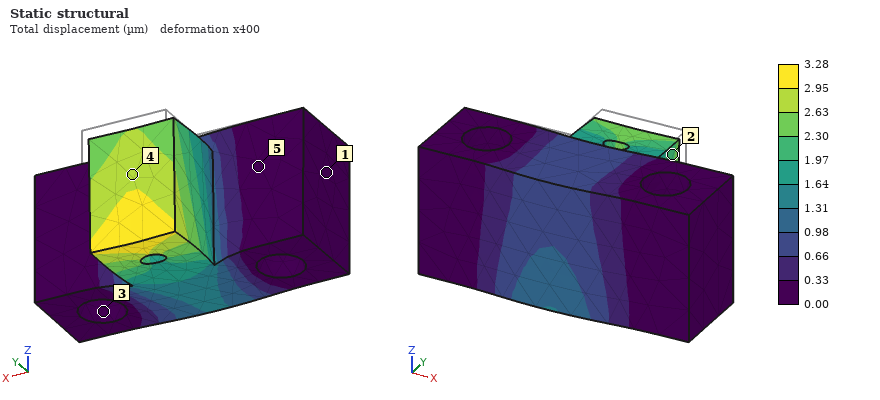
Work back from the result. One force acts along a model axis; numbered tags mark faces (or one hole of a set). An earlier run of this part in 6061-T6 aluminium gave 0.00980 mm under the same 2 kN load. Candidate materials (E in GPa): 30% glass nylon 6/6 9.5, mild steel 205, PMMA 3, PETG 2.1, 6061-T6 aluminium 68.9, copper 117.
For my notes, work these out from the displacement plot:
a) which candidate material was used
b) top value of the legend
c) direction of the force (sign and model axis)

mild steel
3.28 µm
-Y
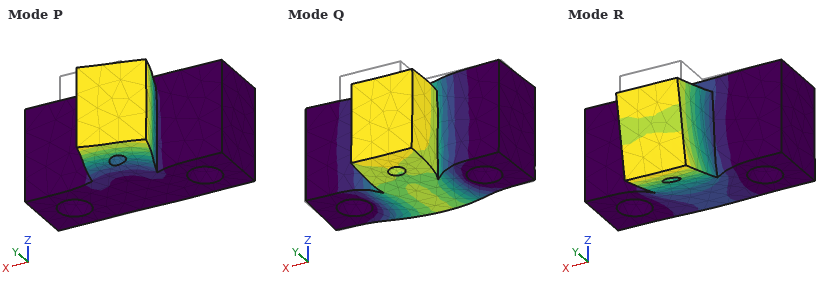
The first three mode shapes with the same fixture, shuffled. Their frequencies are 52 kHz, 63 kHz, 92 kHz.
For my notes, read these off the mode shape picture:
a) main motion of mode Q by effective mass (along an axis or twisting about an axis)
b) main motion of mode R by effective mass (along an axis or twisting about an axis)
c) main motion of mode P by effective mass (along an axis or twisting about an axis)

along Y
along Z
along X
